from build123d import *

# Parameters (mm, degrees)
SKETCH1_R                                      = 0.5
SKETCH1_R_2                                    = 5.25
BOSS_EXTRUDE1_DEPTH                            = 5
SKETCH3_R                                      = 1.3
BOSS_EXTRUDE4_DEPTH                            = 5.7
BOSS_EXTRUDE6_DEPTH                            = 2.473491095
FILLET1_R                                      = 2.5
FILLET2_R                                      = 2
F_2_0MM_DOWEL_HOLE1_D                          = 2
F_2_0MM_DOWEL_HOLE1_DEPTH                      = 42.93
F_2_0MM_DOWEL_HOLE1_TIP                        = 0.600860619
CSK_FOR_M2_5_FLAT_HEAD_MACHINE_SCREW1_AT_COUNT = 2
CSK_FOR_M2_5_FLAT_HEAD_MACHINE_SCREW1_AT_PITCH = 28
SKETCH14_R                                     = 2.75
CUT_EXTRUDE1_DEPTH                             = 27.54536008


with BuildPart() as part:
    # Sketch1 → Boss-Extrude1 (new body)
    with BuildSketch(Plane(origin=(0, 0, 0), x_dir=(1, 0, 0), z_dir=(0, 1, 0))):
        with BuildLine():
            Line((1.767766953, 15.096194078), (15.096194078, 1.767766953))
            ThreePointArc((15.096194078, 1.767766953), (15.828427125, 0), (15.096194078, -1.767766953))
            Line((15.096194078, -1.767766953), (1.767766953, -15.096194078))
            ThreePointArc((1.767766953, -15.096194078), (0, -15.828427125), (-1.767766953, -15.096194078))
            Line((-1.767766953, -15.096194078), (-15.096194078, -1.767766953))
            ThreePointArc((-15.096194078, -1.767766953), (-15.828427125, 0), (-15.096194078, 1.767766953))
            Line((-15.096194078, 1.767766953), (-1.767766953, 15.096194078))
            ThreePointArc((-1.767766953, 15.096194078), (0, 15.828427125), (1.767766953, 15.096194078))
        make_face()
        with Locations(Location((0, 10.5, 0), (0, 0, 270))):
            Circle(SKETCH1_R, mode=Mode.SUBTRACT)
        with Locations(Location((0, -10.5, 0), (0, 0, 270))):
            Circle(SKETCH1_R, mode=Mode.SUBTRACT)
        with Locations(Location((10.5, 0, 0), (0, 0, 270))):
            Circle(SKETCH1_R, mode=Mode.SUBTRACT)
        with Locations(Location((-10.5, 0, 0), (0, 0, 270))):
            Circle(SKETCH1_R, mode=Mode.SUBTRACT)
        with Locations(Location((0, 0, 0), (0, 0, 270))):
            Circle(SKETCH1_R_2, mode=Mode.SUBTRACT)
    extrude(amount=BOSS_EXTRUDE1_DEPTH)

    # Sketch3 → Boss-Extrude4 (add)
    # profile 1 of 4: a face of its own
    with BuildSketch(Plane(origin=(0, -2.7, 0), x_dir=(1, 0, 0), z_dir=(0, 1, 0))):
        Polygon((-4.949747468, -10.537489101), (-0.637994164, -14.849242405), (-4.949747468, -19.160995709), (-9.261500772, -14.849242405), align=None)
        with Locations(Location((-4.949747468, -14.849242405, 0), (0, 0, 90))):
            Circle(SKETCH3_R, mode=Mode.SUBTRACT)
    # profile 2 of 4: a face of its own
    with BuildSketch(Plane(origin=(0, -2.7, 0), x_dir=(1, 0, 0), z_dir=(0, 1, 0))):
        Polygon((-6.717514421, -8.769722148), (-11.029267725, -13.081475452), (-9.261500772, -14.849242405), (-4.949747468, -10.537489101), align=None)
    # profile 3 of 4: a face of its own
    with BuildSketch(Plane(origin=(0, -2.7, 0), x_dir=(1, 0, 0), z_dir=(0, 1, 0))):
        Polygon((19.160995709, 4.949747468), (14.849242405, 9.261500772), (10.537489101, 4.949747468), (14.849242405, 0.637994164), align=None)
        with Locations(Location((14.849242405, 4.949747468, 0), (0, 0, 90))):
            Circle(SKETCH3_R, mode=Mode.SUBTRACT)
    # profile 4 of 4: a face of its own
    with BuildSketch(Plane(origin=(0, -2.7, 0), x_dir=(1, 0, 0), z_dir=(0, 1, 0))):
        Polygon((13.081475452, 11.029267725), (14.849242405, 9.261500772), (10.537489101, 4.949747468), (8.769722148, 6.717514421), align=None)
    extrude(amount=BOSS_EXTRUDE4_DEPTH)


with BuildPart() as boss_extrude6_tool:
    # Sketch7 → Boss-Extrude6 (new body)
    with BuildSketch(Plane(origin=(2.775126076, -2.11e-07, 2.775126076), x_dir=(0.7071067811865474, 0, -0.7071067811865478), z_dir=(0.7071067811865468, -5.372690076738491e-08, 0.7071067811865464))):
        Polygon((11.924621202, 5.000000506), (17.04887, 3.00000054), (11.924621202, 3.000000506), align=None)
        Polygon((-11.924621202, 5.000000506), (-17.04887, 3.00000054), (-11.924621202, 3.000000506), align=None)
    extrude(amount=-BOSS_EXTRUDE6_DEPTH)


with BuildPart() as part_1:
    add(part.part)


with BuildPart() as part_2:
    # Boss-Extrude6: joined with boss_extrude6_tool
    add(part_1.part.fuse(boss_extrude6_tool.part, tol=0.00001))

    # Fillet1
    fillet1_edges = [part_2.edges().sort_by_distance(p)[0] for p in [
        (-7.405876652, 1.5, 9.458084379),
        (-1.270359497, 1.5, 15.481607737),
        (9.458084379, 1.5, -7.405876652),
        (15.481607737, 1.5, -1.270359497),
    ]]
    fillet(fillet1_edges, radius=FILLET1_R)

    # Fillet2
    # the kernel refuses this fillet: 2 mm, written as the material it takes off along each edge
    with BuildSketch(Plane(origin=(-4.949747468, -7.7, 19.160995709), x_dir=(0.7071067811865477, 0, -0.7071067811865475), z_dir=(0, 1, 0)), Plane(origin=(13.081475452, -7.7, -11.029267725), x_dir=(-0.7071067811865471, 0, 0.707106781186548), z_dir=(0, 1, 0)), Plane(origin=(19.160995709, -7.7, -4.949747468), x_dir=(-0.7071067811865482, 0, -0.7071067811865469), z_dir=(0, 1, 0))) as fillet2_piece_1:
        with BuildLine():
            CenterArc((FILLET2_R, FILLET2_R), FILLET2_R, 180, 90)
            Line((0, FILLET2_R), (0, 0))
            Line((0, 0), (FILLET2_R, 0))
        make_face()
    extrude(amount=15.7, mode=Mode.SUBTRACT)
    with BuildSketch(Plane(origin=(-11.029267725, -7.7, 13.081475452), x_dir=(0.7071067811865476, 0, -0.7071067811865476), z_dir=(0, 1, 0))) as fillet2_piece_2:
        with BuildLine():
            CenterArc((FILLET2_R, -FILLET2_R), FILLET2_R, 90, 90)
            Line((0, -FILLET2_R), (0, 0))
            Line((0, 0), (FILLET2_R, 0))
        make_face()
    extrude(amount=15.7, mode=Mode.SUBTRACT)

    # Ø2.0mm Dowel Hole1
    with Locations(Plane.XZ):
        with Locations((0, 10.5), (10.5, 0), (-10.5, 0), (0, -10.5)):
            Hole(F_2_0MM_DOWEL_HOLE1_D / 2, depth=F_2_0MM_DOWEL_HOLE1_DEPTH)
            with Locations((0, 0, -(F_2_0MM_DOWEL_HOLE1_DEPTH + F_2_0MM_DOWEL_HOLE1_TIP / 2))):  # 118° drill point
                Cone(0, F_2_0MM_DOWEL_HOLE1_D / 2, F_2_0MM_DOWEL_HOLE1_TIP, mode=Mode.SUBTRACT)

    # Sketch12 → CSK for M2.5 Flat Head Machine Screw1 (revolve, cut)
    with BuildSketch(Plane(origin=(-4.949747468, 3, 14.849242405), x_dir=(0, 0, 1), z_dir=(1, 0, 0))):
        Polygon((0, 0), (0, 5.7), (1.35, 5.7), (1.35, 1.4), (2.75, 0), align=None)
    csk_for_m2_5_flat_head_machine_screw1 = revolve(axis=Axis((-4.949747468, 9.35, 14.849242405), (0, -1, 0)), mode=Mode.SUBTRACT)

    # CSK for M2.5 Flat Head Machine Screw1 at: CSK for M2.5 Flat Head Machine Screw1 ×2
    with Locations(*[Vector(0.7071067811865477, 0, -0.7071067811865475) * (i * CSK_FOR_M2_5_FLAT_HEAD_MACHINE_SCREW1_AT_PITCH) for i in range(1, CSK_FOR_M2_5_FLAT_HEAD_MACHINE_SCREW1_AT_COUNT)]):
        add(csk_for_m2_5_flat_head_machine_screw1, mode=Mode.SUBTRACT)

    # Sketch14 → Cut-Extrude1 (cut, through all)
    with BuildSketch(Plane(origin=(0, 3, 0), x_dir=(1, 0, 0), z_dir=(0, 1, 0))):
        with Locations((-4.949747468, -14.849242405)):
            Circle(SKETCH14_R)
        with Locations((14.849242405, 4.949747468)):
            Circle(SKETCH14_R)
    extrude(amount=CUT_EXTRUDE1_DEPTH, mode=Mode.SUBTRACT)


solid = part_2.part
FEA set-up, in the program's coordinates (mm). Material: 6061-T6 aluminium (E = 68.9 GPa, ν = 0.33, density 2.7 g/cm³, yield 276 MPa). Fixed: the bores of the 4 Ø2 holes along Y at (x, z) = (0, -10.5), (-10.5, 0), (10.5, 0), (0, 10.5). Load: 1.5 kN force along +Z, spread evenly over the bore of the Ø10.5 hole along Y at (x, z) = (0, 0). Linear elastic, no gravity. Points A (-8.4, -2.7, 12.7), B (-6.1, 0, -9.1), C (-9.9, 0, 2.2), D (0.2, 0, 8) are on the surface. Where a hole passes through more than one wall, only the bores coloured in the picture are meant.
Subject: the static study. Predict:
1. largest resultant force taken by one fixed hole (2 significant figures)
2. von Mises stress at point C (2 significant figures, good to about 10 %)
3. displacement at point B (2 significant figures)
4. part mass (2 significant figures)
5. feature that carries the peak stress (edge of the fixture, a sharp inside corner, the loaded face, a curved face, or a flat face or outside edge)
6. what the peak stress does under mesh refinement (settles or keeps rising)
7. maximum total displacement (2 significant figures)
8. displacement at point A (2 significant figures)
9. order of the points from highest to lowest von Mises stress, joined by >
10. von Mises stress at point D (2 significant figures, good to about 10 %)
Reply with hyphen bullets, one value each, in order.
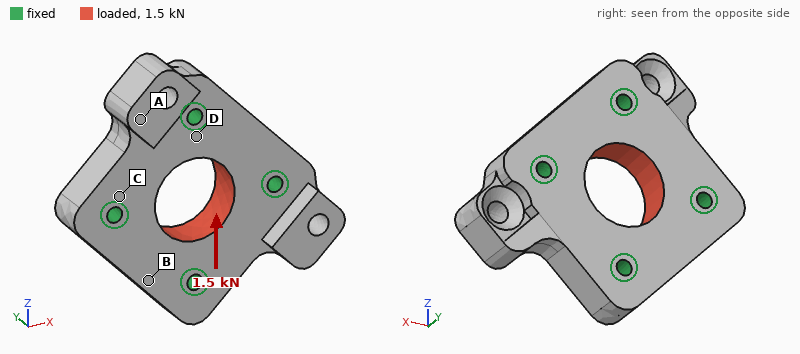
- 450 N
- 9.5 MPa
- 1.0 µm
- 7.5 g
- edge of the fixture
- keeps rising
- 1.7 µm
- 0.97 µm
- D > C > B > A
- 17 MPa
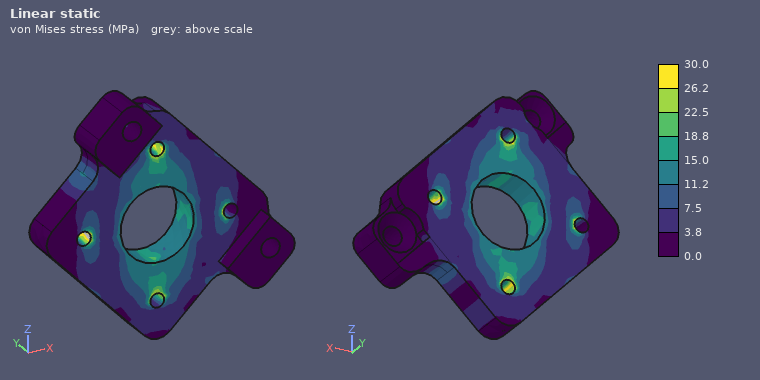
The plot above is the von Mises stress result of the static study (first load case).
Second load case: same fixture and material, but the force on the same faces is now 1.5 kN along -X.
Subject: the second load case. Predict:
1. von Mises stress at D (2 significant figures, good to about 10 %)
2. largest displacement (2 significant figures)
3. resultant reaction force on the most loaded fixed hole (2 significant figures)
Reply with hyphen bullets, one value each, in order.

- 6.5 MPa
- 1.7 µm
- 450 N
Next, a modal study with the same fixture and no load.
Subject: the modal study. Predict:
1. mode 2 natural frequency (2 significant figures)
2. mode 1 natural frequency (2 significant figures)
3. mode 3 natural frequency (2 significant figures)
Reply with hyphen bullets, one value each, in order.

- 32 kHz
- 31 kHz
- 51 kHz
